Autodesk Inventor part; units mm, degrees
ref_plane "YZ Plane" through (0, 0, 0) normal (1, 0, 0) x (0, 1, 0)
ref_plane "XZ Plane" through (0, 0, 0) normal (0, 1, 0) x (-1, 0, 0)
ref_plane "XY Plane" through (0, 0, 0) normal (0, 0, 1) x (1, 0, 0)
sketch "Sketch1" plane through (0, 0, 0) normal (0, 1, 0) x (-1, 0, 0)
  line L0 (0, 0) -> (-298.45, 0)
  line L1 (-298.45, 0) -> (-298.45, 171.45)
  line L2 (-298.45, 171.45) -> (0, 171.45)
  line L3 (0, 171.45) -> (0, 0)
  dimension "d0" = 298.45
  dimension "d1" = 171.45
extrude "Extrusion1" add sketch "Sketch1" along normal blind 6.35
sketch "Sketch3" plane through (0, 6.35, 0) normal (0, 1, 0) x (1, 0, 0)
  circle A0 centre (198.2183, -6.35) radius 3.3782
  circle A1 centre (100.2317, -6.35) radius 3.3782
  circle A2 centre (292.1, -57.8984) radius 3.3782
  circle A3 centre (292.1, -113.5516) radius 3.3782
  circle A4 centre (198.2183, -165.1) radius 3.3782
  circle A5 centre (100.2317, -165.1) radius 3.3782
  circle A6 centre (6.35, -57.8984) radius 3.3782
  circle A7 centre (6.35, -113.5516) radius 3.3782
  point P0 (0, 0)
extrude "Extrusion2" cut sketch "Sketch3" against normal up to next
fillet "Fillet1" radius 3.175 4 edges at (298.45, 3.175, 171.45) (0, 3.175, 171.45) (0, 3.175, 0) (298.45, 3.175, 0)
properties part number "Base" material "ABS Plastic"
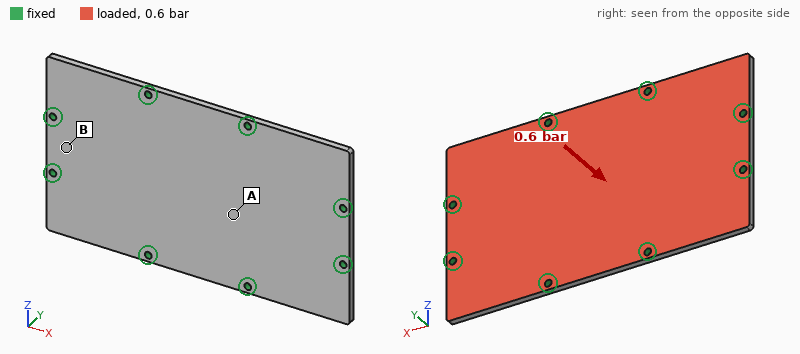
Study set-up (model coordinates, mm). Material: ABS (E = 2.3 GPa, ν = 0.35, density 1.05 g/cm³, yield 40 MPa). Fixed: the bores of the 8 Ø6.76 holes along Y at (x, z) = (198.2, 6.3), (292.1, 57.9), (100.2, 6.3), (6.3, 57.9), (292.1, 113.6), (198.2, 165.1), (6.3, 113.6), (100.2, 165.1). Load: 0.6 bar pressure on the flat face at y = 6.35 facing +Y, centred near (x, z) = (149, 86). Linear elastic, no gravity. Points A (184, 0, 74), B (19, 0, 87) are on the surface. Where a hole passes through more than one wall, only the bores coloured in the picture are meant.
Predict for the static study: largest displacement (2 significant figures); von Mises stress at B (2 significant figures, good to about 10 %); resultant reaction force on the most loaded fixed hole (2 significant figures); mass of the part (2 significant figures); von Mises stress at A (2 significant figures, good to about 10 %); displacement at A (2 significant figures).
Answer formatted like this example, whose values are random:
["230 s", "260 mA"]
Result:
["2.7 mm", "4.4 MPa", "470 N", "340 g", "8.7 MPa", "2.4 mm"]
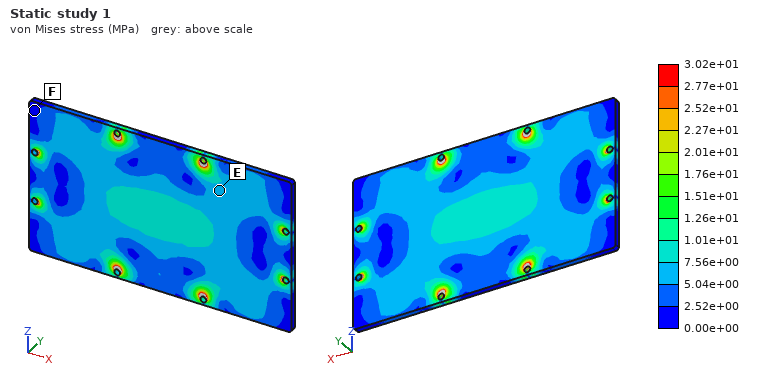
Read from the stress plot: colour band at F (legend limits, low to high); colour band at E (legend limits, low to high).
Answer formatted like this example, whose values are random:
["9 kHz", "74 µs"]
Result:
["0.00e+00 to 2.52e+00 MPa", "5.04e+00 to 7.56e+00 MPa"]
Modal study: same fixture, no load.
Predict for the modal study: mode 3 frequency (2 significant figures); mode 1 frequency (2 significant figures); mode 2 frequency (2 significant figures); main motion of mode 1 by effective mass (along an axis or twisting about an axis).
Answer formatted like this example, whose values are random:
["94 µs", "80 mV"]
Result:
["550 Hz", "350 Hz", "530 Hz", "along Y"]
